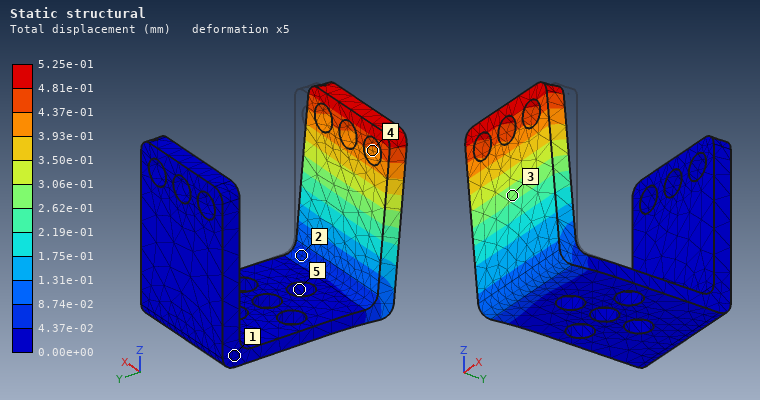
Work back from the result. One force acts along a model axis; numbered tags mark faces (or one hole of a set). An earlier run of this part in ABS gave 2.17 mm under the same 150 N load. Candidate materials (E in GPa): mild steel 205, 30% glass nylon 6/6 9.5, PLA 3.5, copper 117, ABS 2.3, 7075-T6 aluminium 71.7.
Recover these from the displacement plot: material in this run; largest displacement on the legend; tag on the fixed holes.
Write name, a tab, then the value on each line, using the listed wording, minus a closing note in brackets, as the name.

material in this run	30% glass nylon 6/6
largest displacement on the legend	5.25e-01 mm
tag on the fixed holes	5
